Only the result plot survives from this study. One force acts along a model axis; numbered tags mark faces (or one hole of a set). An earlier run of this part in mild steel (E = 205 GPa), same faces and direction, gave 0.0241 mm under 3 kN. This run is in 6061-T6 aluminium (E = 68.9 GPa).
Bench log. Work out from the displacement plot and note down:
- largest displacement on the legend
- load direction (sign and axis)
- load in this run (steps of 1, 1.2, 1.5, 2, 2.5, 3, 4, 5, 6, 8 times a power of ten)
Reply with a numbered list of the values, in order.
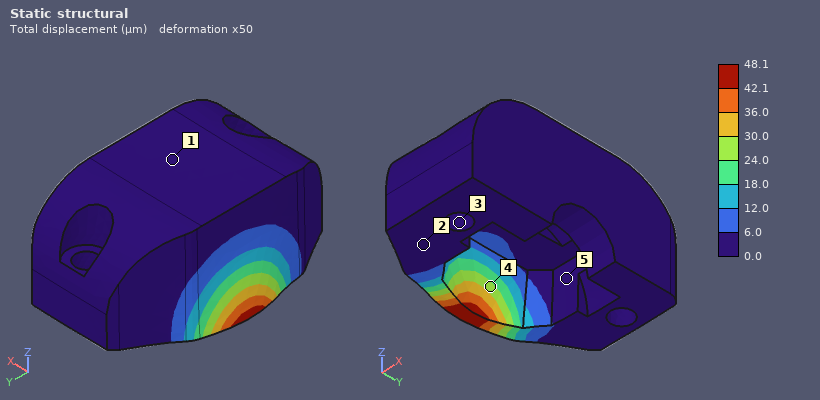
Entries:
1. 48.1 µm
2. -X
3. 2 kN
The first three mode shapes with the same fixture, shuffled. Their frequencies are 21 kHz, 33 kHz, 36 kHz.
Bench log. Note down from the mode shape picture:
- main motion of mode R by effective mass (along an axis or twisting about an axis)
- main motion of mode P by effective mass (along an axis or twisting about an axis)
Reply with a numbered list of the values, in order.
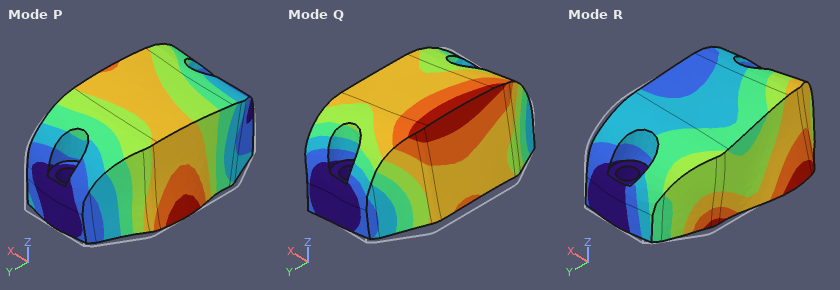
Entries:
1. along Y
2. along Z
